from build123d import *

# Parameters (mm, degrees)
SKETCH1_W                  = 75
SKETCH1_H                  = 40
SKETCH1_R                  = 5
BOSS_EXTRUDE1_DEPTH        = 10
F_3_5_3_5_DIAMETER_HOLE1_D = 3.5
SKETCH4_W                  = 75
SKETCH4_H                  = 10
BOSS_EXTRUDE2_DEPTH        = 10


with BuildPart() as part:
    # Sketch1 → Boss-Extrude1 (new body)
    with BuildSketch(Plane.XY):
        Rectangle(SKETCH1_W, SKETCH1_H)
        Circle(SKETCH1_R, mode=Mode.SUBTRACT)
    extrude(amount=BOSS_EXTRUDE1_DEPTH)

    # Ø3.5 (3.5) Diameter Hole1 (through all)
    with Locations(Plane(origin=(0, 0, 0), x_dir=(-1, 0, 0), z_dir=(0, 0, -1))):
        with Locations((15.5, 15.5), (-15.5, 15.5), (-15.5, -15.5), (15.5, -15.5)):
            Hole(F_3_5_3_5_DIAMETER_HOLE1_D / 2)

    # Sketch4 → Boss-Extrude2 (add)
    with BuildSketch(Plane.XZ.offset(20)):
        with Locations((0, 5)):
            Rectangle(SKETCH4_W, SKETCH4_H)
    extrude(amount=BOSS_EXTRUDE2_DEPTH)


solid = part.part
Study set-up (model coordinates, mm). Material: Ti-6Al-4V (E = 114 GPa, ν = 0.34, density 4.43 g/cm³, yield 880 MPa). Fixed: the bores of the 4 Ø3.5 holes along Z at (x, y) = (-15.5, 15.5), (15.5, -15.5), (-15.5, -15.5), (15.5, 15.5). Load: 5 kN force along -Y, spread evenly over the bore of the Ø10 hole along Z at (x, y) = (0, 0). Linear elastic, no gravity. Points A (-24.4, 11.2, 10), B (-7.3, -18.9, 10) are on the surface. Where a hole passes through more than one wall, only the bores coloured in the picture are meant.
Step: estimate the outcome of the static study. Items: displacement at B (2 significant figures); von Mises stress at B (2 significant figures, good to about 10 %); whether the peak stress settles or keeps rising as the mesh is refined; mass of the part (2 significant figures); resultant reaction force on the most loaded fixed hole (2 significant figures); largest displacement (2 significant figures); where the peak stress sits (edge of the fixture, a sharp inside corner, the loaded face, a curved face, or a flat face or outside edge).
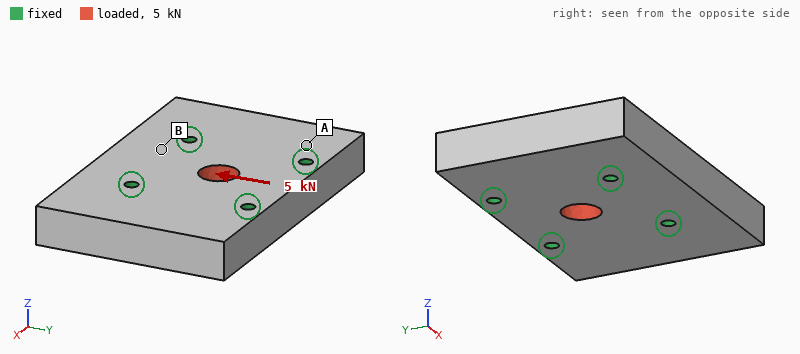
1.0 µm
6.2 MPa
keeps rising
160 g
1.4 kN
2.9 µm
edge of the fixture
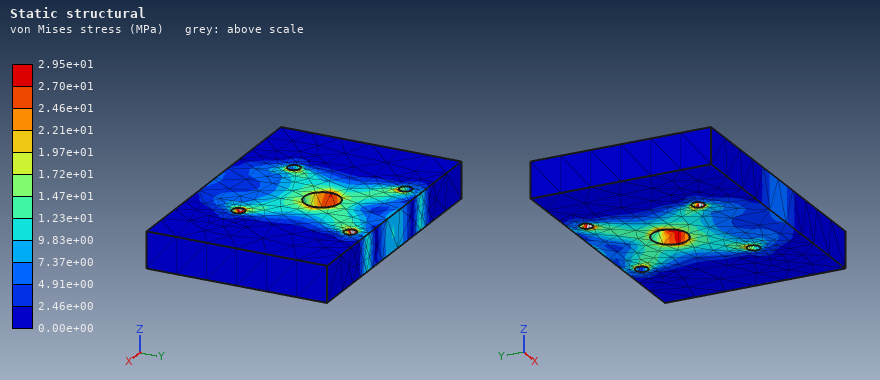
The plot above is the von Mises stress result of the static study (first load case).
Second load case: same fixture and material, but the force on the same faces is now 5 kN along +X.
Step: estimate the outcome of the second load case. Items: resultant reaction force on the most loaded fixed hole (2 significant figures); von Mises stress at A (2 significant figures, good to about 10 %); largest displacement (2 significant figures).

1.3 kN
4.3 MPa
2.3 µm
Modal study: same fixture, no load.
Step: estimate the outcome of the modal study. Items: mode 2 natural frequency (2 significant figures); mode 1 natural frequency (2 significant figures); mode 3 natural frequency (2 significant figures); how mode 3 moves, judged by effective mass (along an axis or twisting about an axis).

12 kHz
12 kHz
17 kHz
twisting about X
